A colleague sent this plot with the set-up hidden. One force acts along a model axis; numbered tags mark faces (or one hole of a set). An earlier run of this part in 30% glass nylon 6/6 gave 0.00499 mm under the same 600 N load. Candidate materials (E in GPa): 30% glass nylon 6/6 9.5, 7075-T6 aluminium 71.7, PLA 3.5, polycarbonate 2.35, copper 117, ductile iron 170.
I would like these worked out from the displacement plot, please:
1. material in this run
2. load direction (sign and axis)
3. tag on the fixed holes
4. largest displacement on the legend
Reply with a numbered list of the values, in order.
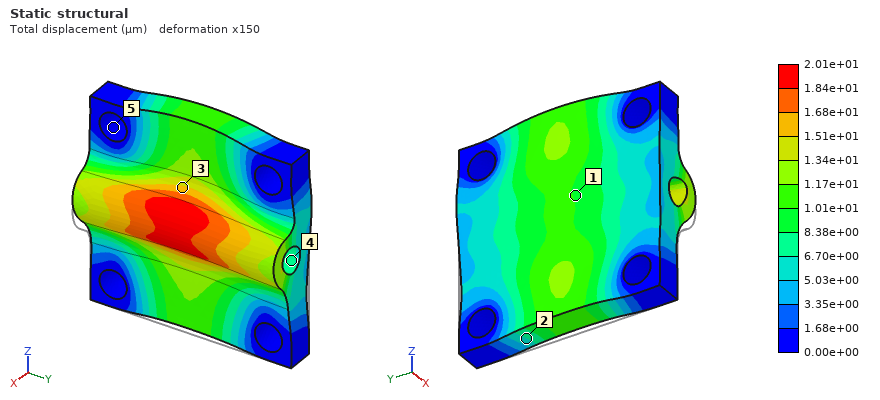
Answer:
1. polycarbonate
2. +Z
3. 5
4. 2.01e+01 µm
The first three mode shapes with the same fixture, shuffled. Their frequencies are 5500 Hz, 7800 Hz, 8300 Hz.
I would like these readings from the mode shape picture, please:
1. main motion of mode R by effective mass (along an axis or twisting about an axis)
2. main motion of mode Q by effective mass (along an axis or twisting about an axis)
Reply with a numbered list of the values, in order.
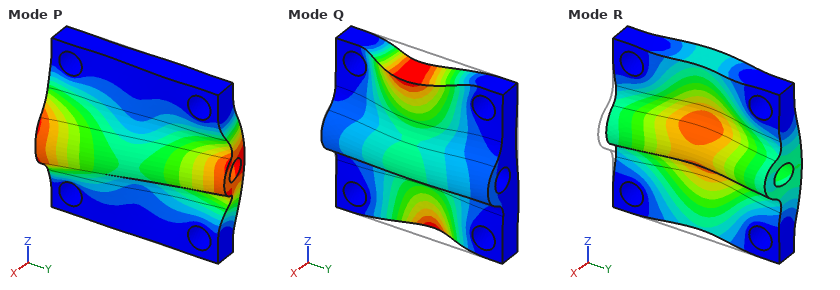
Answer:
1. along X
2. twisting about Y
